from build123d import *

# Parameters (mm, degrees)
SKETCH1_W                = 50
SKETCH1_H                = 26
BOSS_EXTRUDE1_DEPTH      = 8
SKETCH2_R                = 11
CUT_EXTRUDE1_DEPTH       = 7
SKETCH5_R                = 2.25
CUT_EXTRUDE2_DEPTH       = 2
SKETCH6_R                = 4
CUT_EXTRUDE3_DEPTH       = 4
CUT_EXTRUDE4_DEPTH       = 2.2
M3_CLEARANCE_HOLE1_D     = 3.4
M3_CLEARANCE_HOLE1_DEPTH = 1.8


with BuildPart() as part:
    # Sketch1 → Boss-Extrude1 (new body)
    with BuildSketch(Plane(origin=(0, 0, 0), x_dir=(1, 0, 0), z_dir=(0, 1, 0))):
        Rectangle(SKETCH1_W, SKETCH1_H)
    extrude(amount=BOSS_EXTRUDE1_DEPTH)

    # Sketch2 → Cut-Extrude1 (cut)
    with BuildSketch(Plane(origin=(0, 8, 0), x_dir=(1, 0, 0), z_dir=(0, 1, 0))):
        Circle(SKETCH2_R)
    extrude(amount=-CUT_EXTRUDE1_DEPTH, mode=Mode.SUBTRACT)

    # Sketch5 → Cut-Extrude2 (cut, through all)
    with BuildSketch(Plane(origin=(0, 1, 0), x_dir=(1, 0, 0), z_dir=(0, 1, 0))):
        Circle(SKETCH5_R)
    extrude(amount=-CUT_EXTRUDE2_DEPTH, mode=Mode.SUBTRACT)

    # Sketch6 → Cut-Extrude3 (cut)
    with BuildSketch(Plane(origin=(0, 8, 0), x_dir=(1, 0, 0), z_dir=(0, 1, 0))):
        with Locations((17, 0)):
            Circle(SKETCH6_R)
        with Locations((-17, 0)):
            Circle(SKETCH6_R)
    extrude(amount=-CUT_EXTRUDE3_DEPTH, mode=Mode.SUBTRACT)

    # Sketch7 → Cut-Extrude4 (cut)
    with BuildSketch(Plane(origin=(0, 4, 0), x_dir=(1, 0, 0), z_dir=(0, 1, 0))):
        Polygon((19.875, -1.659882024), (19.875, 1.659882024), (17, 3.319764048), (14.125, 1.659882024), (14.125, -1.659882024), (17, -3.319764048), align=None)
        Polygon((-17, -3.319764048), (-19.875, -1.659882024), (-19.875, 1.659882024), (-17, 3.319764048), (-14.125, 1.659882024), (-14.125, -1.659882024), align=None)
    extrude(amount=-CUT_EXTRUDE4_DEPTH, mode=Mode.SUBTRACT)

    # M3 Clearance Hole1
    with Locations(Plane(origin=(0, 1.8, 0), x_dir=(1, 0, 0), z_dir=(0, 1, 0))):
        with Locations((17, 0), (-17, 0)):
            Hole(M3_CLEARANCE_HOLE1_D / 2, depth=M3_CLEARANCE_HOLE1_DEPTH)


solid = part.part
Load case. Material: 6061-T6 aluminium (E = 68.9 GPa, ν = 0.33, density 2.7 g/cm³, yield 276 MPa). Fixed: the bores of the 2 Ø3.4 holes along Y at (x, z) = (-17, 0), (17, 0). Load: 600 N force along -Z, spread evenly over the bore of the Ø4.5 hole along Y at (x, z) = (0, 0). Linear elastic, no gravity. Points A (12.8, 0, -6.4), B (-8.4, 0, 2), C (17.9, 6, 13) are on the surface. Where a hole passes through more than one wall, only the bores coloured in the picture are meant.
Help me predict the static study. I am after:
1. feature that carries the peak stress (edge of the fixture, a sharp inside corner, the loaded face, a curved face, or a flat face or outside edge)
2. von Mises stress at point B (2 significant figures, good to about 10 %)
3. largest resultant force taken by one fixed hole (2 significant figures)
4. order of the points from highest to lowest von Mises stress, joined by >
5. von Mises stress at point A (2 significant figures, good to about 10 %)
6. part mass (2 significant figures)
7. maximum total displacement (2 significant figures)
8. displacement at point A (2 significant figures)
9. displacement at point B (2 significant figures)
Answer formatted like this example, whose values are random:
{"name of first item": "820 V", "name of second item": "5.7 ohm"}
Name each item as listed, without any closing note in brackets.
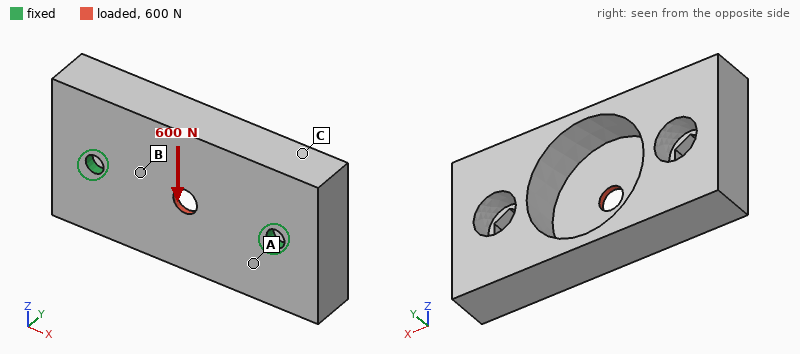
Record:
{"feature that carries the peak stress": "the loaded face", "von Mises stress at point B": "14 MPa", "largest resultant force taken by one fixed hole": "300 N", "order of the points from highest to lowest von Mises stress, joined by >": "B > A > C", "von Mises stress at point A": "7.8 MPa", "part mass": "19 g", "maximum total displacement": "7.7 µm", "displacement at point A": "1.6 µm", "displacement at point B": "2.8 µm"}
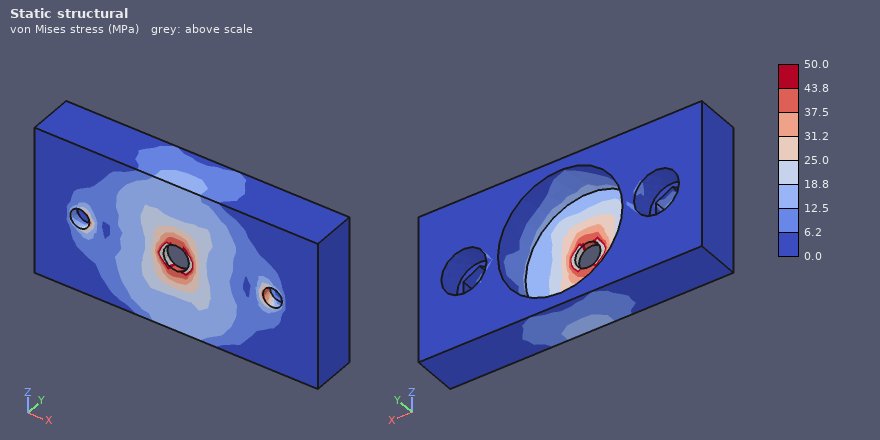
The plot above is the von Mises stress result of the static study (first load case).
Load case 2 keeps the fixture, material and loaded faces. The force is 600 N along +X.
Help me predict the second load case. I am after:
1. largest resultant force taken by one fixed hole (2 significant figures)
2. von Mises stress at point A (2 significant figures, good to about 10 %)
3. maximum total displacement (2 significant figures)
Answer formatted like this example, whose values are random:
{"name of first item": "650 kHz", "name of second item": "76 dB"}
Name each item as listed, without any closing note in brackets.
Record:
{"largest resultant force taken by one fixed hole": "300 N", "von Mises stress at point A": "6.0 MPa", "maximum total displacement": "5.2 µm"}
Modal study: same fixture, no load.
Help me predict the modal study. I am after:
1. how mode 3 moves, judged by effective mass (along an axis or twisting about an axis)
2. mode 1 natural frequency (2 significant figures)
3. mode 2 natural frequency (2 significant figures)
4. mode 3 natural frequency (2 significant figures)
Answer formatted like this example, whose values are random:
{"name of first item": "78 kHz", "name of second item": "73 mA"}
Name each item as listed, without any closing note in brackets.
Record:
{"how mode 3 moves, judged by effective mass": "along Y", "mode 1 natural frequency": "5100 Hz", "mode 2 natural frequency": "11 kHz", "mode 3 natural frequency": "13 kHz"}
